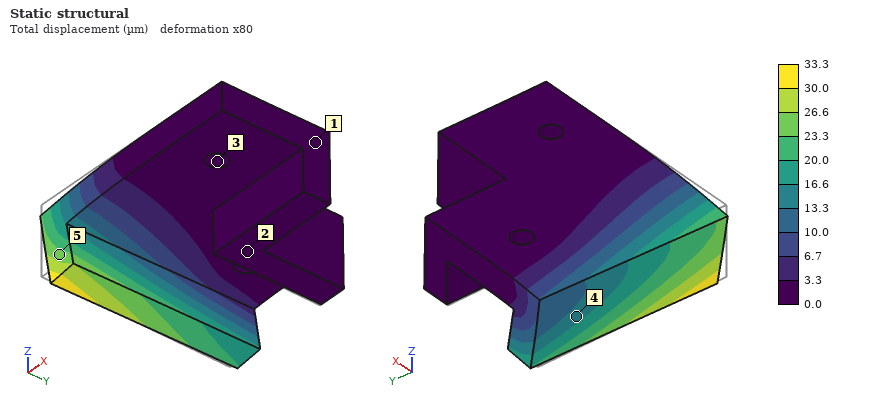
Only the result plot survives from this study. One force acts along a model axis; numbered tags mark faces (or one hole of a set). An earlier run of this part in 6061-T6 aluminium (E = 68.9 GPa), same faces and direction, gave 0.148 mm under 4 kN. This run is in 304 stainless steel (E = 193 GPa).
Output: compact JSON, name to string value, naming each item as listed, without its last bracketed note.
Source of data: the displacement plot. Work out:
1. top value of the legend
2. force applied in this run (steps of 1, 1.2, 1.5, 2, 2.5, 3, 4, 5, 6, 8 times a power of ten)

{"top value of the legend": "33.3 µm", "force applied in this run": "2.5 kN"}
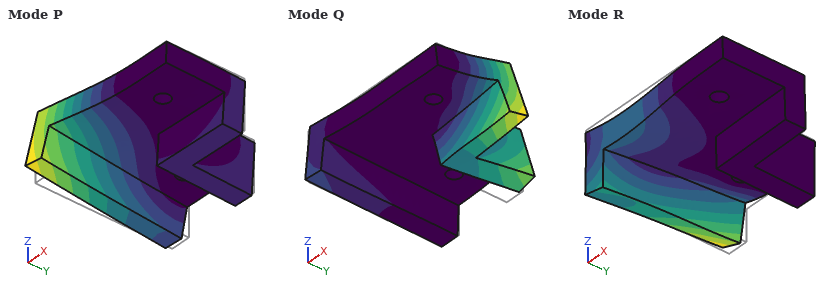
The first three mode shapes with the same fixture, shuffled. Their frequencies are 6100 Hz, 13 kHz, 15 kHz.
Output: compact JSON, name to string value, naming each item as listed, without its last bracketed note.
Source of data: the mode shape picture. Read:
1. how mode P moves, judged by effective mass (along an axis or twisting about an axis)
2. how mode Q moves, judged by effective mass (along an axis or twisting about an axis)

{"how mode P moves, judged by effective mass": "along Z", "how mode Q moves, judged by effective mass": "along Z"}
